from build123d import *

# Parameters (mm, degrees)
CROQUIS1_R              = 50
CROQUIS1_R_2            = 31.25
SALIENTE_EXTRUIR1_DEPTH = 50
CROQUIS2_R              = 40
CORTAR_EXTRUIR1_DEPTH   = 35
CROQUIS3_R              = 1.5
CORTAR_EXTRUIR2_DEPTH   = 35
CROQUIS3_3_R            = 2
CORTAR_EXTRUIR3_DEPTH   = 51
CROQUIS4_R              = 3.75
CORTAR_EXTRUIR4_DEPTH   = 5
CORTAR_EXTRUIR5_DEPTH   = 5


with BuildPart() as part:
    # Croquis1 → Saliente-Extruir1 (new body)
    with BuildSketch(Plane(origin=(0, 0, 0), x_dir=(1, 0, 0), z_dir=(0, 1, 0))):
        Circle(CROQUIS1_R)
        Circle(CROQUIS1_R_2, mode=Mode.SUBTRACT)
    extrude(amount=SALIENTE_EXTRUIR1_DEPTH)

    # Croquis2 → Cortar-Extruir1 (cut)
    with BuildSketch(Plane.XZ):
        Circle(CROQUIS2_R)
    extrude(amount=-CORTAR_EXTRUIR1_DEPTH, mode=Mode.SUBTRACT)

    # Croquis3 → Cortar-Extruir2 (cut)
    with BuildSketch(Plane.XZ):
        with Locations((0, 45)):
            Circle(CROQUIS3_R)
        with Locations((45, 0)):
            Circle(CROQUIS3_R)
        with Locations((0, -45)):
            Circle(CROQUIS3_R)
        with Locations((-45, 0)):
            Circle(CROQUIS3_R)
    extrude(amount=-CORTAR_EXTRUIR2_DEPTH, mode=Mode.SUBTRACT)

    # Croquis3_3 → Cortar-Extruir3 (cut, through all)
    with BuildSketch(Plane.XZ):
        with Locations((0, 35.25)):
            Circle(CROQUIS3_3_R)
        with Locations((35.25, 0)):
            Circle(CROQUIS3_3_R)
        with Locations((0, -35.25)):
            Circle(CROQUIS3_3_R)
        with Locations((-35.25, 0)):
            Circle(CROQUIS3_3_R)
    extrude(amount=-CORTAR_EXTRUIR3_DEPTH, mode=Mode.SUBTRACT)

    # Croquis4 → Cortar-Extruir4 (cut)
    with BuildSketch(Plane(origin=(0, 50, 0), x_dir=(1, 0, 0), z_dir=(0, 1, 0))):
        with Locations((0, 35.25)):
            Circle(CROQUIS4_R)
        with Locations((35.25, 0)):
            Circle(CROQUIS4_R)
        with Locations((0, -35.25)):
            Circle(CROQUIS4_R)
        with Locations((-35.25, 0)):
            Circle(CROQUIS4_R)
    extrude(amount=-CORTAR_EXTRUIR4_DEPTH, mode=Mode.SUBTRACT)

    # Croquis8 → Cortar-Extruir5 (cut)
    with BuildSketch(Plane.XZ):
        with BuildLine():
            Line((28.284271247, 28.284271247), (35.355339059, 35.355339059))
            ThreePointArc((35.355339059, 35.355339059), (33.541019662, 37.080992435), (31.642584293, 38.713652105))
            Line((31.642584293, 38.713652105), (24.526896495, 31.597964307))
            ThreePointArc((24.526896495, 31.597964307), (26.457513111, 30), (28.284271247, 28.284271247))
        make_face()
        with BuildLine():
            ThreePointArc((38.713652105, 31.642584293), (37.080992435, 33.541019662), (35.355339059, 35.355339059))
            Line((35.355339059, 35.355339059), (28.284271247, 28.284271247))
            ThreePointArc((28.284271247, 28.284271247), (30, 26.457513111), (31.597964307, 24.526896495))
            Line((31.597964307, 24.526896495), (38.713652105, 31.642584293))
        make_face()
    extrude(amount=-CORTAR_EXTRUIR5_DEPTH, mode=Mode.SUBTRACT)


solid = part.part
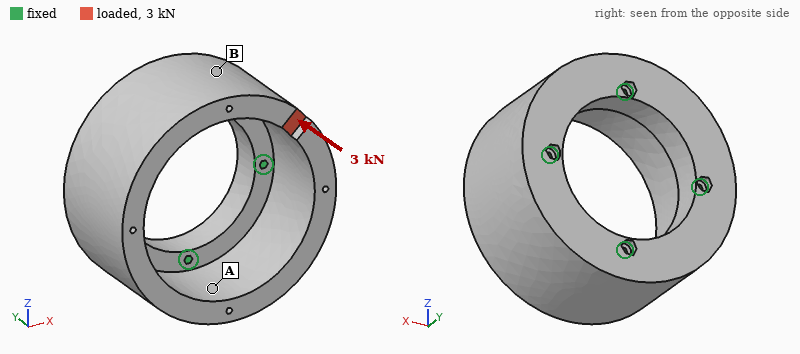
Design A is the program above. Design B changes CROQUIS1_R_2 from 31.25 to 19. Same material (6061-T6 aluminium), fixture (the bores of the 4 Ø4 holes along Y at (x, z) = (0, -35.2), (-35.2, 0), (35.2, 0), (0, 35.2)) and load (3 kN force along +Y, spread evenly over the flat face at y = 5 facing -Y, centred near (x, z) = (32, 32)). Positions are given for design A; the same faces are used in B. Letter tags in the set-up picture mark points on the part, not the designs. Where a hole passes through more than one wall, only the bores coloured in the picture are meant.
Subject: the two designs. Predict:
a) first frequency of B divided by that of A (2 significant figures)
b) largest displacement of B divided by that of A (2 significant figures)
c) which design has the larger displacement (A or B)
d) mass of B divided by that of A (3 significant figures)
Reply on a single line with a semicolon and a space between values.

1.1; 0.89; A; 1.17
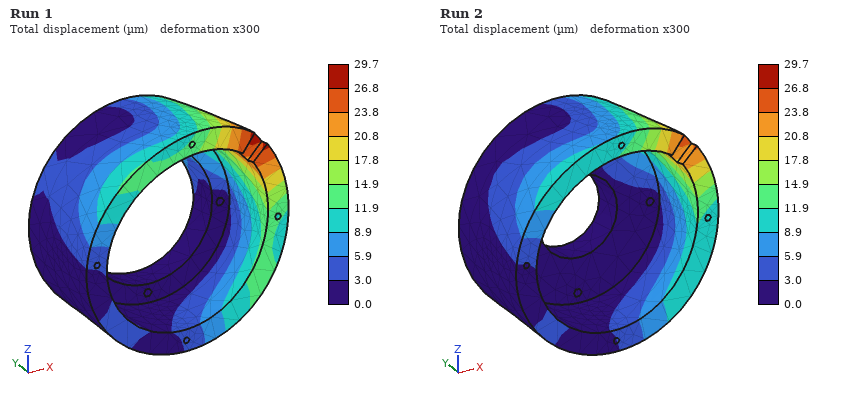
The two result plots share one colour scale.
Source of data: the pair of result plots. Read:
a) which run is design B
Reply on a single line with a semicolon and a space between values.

Run 2
